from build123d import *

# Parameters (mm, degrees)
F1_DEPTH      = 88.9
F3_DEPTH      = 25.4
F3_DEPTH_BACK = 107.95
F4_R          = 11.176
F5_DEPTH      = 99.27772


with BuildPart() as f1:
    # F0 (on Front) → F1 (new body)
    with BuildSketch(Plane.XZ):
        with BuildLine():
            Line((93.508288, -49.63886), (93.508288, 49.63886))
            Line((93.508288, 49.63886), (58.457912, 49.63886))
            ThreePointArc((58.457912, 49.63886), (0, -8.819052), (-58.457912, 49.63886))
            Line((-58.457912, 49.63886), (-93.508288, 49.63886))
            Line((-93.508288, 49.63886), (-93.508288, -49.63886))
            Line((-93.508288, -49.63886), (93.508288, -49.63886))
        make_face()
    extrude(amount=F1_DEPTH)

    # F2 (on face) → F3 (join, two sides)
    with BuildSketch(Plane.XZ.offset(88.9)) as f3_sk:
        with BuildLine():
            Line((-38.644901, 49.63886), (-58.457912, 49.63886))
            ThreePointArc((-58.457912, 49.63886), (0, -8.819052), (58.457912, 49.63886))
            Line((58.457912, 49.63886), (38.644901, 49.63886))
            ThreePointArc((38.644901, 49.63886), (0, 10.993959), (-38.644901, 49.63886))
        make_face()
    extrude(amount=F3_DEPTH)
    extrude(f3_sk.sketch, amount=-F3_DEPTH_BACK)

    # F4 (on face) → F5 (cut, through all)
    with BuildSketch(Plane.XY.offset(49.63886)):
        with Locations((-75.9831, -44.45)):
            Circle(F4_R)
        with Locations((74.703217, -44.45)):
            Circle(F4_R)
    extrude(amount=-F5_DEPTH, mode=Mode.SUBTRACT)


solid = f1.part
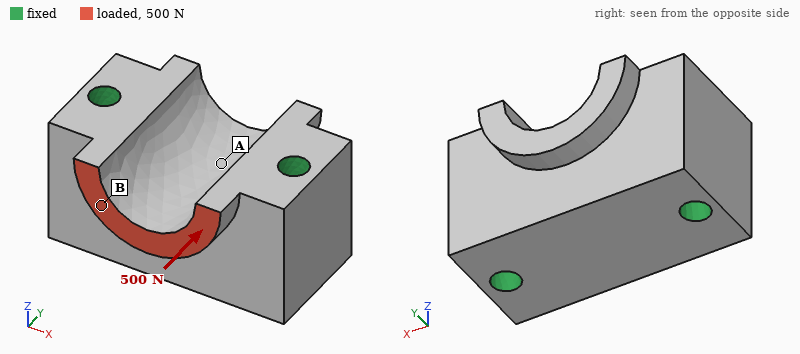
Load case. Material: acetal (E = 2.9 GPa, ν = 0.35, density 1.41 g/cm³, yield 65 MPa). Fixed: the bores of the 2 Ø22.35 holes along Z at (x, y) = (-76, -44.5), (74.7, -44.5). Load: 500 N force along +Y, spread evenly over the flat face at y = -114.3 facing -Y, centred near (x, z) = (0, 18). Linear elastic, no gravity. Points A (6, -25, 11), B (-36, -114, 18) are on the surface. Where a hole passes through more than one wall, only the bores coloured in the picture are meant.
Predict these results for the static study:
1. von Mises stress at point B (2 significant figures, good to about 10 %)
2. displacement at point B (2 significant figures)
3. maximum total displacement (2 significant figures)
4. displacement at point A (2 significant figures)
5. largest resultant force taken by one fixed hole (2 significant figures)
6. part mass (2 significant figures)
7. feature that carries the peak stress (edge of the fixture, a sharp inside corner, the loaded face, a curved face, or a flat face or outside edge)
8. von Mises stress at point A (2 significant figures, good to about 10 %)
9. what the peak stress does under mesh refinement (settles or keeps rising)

0.16 MPa
4.3 µm
6.3 µm
1.8 µm
260 N
2.1 kg
edge of the fixture
0.045 MPa
keeps rising
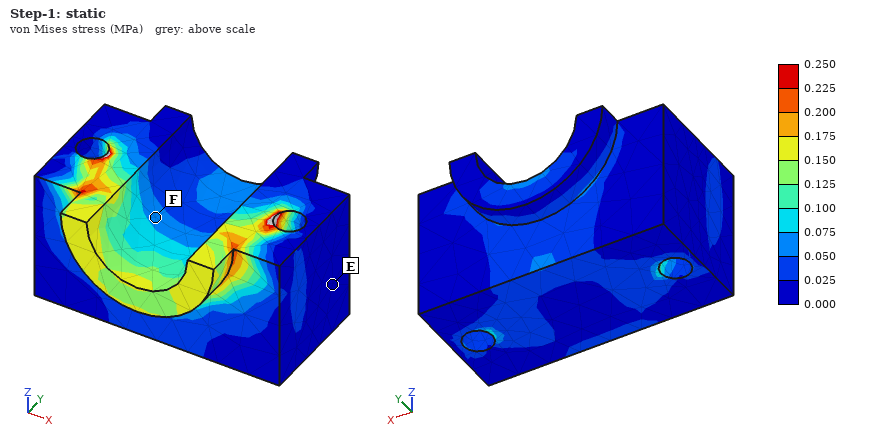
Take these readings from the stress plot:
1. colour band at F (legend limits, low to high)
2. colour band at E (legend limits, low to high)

0.050 to 0.075 MPa
0.000 to 0.025 MPa
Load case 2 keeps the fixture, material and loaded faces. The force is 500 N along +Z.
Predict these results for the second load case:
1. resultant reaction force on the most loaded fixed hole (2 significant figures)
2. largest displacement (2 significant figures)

260 N
26 µm
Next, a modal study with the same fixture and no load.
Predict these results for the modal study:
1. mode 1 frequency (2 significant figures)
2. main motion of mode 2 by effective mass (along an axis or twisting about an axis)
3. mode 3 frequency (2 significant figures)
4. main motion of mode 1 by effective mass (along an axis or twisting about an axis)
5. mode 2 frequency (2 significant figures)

2100 Hz
along Z
2600 Hz
along Y
2300 Hz
